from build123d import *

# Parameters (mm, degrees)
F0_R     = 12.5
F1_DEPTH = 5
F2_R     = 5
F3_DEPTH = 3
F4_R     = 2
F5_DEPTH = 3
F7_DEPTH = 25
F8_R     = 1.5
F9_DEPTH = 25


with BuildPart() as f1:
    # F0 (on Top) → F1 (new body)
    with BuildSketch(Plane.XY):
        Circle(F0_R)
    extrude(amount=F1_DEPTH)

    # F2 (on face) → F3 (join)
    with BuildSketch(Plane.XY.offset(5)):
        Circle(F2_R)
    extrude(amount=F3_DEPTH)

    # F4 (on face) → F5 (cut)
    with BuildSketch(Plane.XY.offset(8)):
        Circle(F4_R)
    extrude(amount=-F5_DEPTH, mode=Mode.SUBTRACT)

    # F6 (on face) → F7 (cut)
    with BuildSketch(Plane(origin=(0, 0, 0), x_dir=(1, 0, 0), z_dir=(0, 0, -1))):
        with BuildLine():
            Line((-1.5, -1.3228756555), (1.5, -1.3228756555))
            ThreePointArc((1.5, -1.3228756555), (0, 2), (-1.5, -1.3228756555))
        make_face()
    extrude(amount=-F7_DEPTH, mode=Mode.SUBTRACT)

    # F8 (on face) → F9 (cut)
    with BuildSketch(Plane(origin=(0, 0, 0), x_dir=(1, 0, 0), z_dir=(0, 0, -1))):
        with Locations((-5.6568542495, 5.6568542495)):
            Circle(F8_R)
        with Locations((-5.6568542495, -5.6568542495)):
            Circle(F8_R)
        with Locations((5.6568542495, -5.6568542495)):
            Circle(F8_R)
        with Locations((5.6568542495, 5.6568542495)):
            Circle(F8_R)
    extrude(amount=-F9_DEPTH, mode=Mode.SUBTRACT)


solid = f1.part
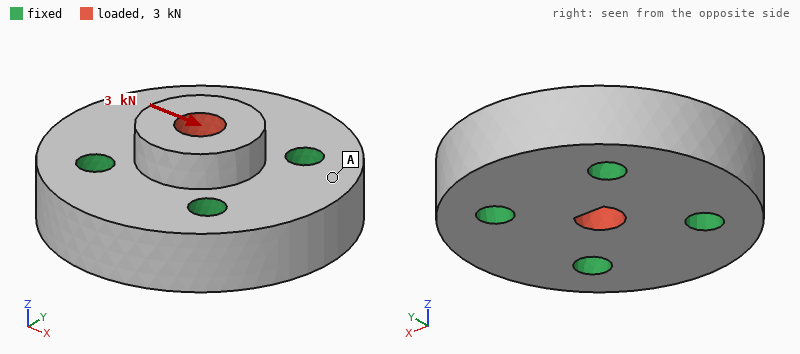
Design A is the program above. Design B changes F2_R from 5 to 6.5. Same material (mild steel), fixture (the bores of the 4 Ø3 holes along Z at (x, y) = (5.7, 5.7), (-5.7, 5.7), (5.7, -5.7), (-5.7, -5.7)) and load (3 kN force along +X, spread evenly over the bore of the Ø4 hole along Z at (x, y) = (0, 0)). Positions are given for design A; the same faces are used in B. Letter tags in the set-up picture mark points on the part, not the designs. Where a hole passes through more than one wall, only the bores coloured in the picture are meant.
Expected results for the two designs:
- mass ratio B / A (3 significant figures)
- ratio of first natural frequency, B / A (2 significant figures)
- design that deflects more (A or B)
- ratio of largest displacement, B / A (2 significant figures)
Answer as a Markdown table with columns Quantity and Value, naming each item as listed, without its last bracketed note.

| Quantity | Value |
|---|---|
| mass ratio B / A | 1.07 |
| ratio of first natural frequency, B / A | 1.0 |
| design that deflects more | A |
| ratio of largest displacement, B / A | 0.68 |
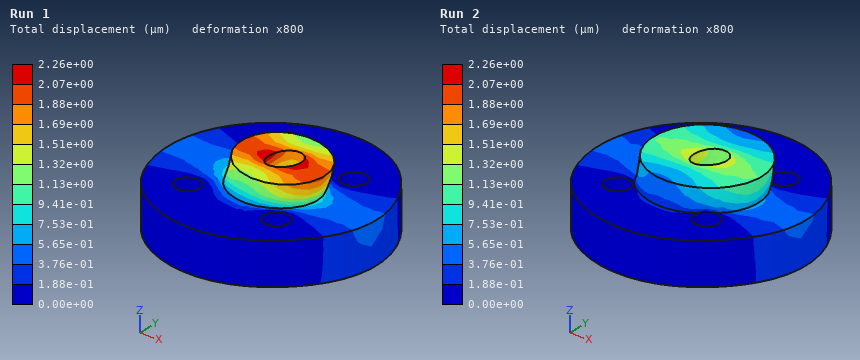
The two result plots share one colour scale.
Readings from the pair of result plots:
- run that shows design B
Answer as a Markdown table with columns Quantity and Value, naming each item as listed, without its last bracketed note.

| Quantity | Value |
|---|---|
| run that shows design B | Run 2 |
